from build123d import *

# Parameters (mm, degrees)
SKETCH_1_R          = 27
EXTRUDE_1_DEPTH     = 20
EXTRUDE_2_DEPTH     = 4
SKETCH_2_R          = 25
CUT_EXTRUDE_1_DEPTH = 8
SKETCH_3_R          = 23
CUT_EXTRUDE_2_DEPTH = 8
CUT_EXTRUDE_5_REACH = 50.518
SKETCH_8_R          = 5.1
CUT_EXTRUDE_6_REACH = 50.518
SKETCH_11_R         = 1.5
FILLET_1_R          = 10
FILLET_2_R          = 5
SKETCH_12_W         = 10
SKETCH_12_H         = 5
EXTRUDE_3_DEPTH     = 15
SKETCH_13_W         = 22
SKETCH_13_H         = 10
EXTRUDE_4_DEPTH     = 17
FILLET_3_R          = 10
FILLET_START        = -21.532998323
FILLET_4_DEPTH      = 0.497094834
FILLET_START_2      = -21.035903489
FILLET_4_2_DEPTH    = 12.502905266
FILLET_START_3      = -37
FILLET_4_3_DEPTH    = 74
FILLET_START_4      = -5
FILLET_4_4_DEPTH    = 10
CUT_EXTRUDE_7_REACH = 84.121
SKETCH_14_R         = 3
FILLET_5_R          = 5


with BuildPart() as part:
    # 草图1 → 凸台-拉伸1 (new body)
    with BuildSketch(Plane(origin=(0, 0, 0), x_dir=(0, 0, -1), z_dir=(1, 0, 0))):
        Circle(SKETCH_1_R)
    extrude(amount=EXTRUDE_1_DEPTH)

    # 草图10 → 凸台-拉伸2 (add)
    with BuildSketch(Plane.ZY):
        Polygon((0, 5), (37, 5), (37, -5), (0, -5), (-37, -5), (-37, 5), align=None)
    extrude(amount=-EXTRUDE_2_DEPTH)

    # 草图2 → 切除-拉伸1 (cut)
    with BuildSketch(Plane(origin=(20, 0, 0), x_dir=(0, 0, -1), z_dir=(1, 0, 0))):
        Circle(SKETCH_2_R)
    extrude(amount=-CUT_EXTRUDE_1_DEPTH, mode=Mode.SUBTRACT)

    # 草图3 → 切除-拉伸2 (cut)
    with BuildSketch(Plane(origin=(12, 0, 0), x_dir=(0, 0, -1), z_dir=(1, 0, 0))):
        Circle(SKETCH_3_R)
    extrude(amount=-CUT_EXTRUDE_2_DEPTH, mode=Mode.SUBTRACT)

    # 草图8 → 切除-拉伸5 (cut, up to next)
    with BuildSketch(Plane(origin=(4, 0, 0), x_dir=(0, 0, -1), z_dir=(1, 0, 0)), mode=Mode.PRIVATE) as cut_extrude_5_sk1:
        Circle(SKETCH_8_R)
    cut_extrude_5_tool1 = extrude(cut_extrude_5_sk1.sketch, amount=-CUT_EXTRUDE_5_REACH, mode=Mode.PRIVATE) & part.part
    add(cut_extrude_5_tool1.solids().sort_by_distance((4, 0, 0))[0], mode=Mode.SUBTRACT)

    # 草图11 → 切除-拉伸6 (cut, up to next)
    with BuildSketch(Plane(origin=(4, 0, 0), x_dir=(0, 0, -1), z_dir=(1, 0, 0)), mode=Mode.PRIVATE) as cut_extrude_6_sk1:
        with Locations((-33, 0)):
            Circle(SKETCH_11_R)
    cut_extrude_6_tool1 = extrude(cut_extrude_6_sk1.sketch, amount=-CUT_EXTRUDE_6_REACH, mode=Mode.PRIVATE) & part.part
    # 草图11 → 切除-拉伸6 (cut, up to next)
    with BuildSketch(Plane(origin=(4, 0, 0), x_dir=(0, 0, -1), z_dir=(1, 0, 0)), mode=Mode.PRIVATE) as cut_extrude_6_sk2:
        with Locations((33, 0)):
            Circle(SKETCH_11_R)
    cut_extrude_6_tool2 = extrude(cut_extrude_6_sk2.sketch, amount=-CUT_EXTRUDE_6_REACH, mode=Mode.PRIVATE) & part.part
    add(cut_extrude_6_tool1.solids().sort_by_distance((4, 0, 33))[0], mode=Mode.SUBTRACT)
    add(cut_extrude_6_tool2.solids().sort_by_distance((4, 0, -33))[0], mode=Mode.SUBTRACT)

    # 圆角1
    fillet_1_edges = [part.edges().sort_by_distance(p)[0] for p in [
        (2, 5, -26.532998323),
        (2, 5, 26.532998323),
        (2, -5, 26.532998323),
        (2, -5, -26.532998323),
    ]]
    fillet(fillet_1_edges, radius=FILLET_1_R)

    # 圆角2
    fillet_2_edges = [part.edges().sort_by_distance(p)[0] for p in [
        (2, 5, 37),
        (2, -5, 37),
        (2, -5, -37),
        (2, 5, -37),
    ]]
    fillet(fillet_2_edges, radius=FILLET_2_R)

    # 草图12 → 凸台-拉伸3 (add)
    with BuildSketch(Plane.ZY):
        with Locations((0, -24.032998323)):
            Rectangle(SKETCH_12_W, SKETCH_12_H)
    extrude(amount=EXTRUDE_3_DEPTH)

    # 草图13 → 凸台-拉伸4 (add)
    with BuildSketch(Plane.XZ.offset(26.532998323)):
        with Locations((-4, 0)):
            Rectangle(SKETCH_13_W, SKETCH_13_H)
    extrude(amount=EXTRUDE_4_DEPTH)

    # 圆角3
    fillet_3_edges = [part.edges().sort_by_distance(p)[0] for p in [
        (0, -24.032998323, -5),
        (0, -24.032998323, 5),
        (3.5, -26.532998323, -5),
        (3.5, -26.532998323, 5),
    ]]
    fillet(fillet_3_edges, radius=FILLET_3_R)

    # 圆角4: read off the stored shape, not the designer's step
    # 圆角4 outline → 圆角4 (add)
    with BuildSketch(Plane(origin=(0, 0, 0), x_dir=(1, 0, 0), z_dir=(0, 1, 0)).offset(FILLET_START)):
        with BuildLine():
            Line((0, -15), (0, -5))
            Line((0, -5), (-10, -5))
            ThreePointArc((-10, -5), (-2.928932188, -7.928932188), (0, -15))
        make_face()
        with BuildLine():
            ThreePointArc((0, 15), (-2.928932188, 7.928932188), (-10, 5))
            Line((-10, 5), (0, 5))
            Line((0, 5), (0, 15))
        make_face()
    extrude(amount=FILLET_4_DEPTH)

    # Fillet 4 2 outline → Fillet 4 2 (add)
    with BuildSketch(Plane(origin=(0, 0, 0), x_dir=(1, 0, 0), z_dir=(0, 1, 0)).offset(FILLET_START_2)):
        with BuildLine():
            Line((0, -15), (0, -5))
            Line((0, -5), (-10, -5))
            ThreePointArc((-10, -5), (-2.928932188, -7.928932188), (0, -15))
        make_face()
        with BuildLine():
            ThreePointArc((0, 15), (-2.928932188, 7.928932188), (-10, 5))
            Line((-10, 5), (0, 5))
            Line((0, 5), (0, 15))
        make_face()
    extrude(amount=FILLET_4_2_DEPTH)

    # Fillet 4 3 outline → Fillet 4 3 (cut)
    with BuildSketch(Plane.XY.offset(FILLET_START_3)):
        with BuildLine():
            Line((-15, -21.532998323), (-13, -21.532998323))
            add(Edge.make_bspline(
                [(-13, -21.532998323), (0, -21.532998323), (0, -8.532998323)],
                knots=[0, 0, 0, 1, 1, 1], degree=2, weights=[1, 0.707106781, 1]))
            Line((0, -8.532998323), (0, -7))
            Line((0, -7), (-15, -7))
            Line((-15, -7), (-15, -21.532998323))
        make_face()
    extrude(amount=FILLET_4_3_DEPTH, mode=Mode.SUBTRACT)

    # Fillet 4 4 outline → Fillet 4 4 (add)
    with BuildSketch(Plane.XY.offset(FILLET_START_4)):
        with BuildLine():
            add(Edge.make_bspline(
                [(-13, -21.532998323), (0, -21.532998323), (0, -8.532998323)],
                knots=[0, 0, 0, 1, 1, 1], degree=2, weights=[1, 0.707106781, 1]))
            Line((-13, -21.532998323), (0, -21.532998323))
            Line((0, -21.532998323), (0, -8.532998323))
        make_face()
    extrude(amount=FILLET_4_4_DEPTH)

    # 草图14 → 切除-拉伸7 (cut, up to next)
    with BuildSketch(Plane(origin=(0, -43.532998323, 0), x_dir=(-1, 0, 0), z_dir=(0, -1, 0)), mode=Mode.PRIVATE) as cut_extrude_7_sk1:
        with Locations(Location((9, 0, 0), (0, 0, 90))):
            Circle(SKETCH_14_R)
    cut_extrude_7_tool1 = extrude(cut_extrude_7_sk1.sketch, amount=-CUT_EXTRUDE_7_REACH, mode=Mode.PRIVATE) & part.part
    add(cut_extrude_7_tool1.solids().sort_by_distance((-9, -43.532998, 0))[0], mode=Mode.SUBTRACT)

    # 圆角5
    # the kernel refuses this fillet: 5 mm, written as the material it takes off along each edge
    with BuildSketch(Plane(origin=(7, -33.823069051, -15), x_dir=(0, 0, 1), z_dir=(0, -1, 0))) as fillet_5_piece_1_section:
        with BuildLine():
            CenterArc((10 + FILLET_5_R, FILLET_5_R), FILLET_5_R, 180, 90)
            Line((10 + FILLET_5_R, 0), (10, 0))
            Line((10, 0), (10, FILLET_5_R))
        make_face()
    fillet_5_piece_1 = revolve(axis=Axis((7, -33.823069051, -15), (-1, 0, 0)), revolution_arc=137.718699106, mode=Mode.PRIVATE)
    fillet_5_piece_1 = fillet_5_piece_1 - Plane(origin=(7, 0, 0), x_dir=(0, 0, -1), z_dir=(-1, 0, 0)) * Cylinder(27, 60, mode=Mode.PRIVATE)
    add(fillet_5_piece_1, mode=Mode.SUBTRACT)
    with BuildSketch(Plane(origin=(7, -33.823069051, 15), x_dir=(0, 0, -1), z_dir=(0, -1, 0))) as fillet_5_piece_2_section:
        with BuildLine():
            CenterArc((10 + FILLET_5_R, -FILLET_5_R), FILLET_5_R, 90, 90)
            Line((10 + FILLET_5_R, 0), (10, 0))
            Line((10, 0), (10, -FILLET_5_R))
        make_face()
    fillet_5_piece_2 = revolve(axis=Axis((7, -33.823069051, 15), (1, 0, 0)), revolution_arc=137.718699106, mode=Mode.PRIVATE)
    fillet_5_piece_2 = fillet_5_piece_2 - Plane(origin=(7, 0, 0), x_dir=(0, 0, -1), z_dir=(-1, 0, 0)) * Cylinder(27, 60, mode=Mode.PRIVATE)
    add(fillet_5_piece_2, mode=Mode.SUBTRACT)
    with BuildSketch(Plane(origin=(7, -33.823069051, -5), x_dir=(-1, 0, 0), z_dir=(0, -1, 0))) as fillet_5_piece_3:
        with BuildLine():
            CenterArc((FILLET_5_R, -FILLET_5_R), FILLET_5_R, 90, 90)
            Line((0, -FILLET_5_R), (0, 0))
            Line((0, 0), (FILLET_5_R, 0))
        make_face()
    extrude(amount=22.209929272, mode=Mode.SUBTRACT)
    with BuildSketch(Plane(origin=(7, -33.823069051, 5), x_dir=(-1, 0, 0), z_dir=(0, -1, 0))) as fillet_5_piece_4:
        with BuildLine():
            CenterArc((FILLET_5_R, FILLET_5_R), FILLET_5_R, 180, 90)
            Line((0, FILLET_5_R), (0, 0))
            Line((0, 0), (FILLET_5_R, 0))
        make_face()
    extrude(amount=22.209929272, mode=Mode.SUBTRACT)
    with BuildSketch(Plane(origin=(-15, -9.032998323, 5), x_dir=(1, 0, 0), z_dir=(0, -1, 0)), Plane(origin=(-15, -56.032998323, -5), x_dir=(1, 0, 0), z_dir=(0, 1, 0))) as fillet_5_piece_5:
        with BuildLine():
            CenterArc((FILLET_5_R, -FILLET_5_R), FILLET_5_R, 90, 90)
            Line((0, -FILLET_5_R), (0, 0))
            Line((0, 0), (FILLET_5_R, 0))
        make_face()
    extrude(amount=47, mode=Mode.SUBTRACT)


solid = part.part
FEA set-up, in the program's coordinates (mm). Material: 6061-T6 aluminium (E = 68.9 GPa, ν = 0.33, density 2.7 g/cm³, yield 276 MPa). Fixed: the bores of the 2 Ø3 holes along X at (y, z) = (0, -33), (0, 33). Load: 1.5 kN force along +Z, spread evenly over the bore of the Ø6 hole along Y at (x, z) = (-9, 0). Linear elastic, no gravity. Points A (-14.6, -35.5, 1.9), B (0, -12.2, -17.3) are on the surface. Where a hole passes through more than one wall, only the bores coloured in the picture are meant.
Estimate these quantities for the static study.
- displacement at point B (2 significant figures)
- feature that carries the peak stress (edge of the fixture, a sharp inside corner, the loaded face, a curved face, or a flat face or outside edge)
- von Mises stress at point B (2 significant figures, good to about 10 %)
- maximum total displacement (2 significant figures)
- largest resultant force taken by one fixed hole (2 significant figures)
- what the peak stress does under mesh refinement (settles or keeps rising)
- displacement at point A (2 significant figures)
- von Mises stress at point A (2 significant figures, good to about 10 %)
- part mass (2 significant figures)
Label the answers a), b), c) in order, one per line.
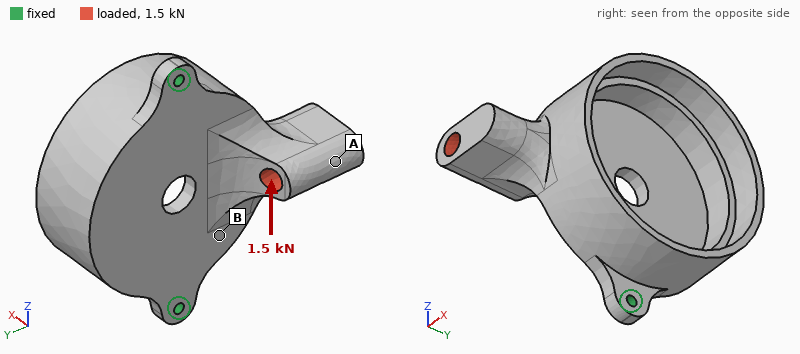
a) 23 µm
b) edge of the fixture
c) 41 MPa
d) 92 µm
e) 1.1 kN
f) keeps rising
g) 78 µm
h) 14 MPa
i) 59 g
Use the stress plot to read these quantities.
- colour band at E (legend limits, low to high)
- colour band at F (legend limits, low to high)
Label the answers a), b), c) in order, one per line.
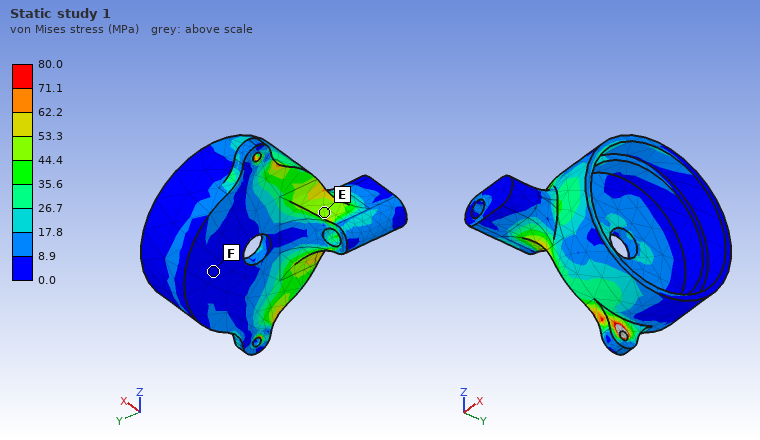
a) 44.4 to 53.3 MPa
b) 0.0 to 8.9 MPa
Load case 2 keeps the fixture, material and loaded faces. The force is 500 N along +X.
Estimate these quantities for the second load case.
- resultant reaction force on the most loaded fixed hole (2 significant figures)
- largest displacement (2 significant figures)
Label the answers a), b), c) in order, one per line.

a) 250 N
b) 0.57 mm
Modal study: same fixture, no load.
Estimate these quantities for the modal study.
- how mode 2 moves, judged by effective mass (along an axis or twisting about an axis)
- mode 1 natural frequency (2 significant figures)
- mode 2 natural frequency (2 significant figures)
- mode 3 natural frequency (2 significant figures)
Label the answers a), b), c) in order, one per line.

a) along X
b) 1200 Hz
c) 3200 Hz
d) 6700 Hz
